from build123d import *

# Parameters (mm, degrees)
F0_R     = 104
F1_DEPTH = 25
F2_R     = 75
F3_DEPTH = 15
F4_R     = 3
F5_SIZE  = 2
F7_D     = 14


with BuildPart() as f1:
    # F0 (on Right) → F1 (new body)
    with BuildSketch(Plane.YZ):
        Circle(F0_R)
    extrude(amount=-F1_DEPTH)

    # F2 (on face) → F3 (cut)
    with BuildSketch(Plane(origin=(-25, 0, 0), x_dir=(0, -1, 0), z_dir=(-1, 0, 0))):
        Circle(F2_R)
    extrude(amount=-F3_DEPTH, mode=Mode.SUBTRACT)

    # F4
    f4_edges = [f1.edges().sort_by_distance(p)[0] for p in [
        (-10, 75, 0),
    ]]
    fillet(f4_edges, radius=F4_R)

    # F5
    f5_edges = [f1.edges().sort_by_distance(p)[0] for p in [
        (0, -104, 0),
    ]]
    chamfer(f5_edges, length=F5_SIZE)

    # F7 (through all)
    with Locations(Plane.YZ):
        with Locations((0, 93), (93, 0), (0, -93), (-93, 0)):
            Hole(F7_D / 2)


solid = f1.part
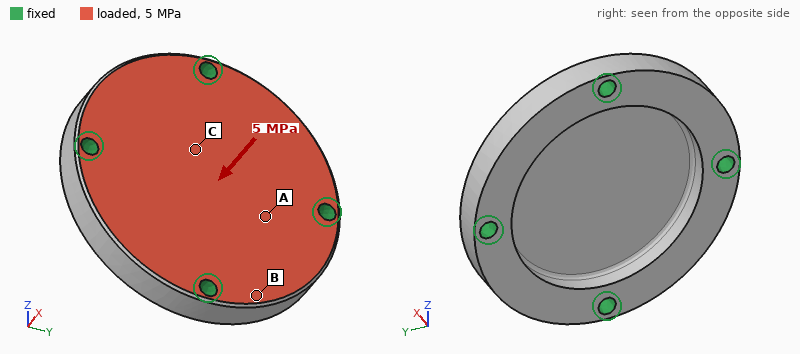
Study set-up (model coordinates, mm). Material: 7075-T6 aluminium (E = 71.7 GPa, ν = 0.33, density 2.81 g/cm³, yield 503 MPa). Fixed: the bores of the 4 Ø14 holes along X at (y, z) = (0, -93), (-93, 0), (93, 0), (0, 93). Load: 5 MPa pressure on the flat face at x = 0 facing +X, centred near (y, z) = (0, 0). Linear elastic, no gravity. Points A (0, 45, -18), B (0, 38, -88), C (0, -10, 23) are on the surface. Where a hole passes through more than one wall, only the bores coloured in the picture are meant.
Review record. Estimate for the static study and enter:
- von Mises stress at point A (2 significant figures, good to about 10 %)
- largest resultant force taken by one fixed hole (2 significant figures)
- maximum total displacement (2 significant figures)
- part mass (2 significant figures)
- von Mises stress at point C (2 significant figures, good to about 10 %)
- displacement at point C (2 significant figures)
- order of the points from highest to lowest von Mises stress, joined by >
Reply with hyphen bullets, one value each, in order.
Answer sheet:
- 79 MPa
- 42 kN
- 0.61 mm
- 1.6 kg
- 140 MPa
- 0.52 mm
- C > A > B
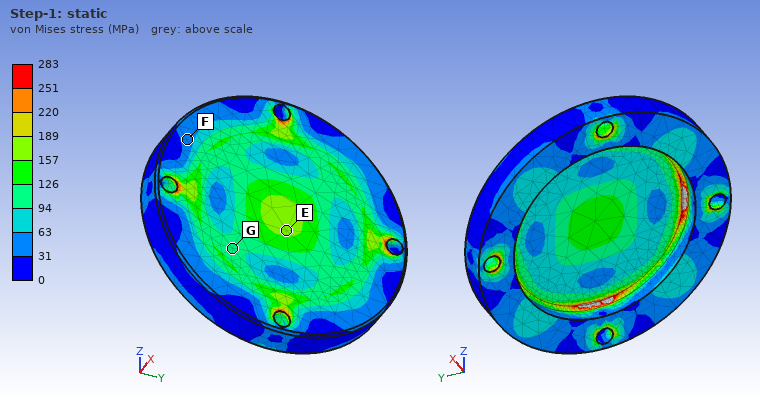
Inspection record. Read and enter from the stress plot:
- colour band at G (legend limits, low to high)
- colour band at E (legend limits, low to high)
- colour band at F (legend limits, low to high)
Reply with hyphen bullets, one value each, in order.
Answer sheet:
- 94 to 126 MPa
- 157 to 189 MPa
- 31 to 63 MPa
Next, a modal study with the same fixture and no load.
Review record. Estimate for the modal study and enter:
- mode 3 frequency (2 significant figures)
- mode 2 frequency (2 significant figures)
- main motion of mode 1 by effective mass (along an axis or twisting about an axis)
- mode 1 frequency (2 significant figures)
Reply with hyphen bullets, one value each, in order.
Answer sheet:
- 5400 Hz
- 5300 Hz
- along X
- 3400 Hz
